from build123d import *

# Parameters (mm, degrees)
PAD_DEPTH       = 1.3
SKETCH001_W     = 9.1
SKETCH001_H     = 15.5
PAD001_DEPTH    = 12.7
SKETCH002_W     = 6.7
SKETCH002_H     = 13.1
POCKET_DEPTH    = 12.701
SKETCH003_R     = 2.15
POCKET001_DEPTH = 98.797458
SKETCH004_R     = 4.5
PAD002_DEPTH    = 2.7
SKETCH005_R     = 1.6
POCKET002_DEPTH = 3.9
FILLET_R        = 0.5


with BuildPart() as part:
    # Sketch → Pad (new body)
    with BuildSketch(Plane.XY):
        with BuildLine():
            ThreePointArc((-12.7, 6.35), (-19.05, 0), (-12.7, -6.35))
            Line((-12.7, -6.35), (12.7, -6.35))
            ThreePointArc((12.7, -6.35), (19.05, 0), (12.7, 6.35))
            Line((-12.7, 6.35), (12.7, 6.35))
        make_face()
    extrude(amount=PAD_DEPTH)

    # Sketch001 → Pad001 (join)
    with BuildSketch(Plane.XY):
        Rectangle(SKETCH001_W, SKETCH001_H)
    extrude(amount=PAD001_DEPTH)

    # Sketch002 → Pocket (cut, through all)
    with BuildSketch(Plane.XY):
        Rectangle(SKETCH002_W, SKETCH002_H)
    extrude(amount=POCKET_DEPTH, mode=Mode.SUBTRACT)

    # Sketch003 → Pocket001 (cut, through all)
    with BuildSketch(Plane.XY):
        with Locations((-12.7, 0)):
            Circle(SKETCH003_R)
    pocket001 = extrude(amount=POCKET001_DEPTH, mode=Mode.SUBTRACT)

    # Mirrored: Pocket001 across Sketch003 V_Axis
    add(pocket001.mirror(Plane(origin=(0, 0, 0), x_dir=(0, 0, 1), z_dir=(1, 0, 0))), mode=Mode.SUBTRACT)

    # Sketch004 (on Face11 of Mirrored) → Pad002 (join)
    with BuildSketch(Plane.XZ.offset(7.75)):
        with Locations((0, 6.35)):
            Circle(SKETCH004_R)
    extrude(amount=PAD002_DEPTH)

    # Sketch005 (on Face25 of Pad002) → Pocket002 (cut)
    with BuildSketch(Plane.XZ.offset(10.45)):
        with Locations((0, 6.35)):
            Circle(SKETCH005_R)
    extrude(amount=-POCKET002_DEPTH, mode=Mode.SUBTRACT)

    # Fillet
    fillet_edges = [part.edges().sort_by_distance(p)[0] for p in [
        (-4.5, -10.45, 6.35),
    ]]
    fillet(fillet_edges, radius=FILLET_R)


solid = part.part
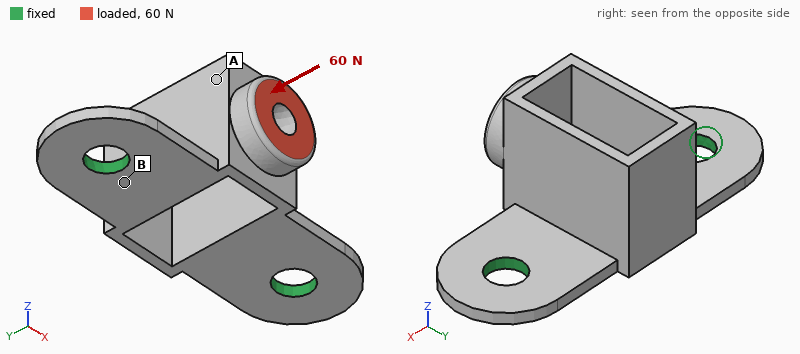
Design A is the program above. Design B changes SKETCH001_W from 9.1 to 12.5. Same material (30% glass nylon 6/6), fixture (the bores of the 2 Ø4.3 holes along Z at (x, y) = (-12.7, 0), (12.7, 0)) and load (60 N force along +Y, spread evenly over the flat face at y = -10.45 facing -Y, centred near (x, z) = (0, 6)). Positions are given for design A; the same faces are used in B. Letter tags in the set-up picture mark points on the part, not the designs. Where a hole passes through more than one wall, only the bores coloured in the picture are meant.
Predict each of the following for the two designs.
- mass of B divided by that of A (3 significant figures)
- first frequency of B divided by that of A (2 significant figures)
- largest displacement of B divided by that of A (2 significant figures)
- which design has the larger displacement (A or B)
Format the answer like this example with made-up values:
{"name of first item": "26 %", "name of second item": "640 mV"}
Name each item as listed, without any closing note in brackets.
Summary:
{"mass of B divided by that of A": "1.51", "first frequency of B divided by that of A": "0.99", "largest displacement of B divided by that of A": "0.63", "which design has the larger displacement": "A"}
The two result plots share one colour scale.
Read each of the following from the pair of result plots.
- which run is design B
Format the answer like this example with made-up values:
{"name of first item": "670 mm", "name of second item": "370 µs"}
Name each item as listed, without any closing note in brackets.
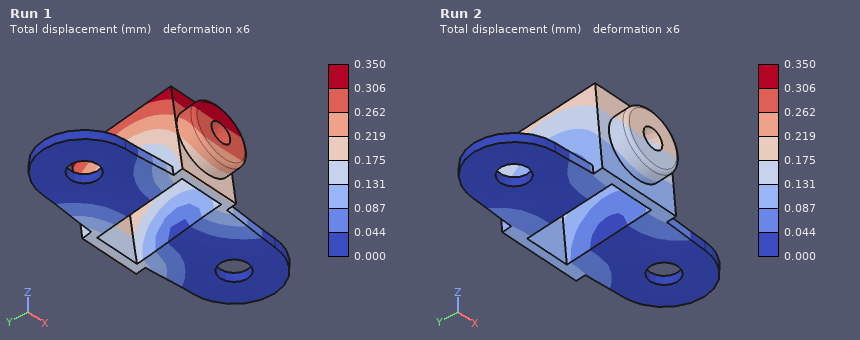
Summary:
{"which run is design B": "Run 2"}
